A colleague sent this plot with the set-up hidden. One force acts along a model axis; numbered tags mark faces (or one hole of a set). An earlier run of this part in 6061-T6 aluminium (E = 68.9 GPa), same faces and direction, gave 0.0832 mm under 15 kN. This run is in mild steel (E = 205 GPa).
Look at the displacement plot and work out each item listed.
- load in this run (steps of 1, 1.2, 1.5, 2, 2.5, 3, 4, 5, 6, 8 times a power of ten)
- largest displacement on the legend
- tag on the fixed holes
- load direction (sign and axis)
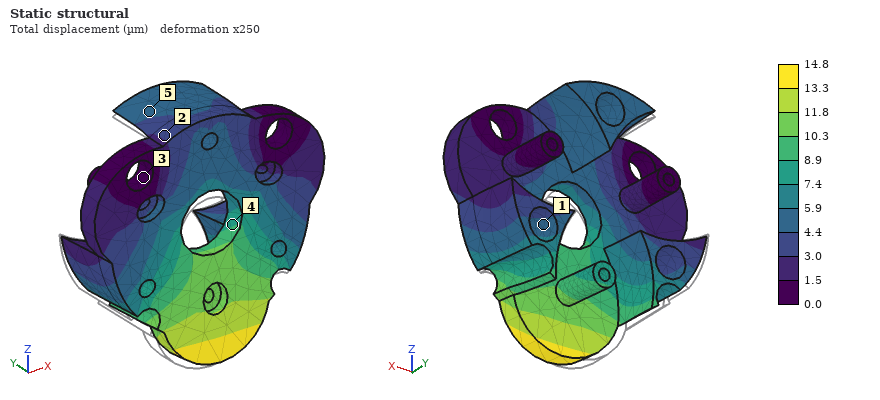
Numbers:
8 kN
14.8 µm
3
+Z
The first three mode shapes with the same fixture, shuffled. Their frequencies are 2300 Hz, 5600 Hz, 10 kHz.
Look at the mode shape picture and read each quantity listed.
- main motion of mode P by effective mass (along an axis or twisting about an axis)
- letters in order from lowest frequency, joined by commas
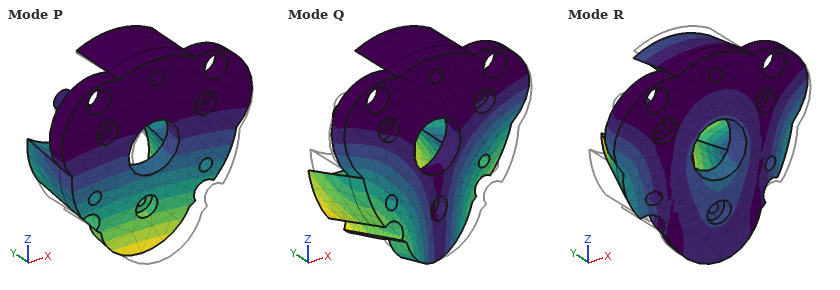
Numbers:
along Y
P, Q, R
